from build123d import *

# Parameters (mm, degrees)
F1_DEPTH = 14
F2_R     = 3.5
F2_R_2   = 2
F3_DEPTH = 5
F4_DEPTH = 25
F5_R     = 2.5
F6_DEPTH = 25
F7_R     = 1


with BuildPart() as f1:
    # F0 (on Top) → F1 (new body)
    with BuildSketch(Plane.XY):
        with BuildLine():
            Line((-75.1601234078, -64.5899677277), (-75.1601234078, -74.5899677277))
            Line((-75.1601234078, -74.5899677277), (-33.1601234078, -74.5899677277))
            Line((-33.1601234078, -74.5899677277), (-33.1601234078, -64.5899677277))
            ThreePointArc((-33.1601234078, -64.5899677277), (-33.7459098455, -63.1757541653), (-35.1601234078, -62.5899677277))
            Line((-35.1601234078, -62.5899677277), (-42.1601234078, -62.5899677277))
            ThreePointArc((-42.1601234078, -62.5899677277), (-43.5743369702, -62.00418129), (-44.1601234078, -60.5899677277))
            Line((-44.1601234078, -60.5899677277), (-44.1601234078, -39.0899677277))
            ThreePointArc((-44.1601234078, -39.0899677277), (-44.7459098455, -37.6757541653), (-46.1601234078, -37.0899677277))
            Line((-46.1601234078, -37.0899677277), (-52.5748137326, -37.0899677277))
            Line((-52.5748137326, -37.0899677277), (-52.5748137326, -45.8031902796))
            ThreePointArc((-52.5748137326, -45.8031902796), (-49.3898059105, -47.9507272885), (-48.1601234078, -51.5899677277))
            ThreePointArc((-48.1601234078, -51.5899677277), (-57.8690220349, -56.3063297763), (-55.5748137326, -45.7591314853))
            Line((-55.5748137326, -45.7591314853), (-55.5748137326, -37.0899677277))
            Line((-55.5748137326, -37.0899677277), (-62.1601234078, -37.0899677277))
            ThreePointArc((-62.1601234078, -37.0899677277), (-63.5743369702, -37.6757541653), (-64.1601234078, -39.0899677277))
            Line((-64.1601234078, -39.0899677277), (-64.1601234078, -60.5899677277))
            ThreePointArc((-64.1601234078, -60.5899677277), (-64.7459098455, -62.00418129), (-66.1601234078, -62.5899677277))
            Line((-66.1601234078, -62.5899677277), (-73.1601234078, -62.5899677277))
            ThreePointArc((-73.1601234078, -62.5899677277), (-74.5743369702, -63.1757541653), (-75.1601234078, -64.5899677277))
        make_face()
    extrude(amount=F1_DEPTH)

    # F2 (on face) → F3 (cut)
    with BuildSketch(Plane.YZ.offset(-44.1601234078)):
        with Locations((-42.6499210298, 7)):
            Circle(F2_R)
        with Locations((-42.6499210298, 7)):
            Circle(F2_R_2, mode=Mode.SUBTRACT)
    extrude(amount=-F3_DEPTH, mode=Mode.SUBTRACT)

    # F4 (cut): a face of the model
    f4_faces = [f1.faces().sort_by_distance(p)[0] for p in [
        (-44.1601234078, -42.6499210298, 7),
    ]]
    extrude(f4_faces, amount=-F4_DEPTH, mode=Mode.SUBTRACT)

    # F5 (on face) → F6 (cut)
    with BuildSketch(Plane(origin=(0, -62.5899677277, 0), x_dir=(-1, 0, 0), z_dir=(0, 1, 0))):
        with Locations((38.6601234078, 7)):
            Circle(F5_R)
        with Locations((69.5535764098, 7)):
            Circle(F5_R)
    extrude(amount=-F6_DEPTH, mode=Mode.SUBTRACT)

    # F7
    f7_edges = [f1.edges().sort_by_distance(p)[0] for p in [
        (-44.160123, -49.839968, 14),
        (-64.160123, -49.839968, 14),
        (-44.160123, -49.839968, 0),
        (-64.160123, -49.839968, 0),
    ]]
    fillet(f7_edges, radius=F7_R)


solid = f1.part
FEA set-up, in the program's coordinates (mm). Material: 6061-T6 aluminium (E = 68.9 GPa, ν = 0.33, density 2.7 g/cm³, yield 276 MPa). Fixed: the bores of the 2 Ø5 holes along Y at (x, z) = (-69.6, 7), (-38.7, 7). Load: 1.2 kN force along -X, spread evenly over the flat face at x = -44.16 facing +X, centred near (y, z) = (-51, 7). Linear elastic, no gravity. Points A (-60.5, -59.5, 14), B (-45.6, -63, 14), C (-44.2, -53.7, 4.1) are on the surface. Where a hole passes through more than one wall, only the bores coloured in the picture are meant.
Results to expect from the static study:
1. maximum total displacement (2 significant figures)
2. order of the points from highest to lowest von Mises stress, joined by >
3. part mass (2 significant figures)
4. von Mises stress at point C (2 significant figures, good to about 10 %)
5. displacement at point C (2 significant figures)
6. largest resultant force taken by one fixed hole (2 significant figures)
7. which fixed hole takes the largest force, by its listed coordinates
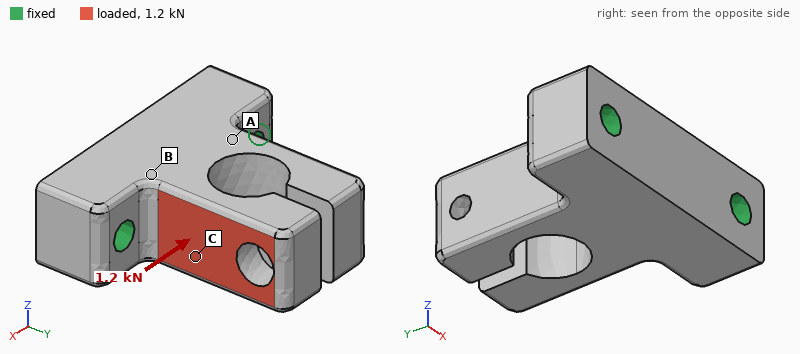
0.13 mm
C > B > A
31 g
97 MPa
0.020 mm
1.0 kN
(-69.6, 7)
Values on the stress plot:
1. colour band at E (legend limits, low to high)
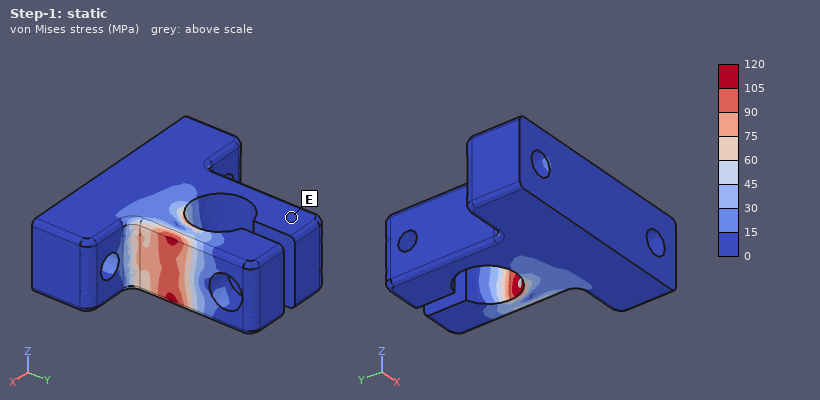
0 to 15 MPa
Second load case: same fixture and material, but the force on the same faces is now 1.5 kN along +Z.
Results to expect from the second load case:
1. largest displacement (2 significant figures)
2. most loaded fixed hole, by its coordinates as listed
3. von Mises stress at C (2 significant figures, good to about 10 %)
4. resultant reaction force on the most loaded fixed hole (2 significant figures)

86 µm
(-38.7, 7)
51 MPa
1.3 kN
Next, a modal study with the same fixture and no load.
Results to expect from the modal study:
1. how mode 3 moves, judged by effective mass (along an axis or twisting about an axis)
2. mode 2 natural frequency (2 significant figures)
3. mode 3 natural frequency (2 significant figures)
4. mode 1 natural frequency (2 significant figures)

along Z
6500 Hz
8200 Hz
6100 Hz
